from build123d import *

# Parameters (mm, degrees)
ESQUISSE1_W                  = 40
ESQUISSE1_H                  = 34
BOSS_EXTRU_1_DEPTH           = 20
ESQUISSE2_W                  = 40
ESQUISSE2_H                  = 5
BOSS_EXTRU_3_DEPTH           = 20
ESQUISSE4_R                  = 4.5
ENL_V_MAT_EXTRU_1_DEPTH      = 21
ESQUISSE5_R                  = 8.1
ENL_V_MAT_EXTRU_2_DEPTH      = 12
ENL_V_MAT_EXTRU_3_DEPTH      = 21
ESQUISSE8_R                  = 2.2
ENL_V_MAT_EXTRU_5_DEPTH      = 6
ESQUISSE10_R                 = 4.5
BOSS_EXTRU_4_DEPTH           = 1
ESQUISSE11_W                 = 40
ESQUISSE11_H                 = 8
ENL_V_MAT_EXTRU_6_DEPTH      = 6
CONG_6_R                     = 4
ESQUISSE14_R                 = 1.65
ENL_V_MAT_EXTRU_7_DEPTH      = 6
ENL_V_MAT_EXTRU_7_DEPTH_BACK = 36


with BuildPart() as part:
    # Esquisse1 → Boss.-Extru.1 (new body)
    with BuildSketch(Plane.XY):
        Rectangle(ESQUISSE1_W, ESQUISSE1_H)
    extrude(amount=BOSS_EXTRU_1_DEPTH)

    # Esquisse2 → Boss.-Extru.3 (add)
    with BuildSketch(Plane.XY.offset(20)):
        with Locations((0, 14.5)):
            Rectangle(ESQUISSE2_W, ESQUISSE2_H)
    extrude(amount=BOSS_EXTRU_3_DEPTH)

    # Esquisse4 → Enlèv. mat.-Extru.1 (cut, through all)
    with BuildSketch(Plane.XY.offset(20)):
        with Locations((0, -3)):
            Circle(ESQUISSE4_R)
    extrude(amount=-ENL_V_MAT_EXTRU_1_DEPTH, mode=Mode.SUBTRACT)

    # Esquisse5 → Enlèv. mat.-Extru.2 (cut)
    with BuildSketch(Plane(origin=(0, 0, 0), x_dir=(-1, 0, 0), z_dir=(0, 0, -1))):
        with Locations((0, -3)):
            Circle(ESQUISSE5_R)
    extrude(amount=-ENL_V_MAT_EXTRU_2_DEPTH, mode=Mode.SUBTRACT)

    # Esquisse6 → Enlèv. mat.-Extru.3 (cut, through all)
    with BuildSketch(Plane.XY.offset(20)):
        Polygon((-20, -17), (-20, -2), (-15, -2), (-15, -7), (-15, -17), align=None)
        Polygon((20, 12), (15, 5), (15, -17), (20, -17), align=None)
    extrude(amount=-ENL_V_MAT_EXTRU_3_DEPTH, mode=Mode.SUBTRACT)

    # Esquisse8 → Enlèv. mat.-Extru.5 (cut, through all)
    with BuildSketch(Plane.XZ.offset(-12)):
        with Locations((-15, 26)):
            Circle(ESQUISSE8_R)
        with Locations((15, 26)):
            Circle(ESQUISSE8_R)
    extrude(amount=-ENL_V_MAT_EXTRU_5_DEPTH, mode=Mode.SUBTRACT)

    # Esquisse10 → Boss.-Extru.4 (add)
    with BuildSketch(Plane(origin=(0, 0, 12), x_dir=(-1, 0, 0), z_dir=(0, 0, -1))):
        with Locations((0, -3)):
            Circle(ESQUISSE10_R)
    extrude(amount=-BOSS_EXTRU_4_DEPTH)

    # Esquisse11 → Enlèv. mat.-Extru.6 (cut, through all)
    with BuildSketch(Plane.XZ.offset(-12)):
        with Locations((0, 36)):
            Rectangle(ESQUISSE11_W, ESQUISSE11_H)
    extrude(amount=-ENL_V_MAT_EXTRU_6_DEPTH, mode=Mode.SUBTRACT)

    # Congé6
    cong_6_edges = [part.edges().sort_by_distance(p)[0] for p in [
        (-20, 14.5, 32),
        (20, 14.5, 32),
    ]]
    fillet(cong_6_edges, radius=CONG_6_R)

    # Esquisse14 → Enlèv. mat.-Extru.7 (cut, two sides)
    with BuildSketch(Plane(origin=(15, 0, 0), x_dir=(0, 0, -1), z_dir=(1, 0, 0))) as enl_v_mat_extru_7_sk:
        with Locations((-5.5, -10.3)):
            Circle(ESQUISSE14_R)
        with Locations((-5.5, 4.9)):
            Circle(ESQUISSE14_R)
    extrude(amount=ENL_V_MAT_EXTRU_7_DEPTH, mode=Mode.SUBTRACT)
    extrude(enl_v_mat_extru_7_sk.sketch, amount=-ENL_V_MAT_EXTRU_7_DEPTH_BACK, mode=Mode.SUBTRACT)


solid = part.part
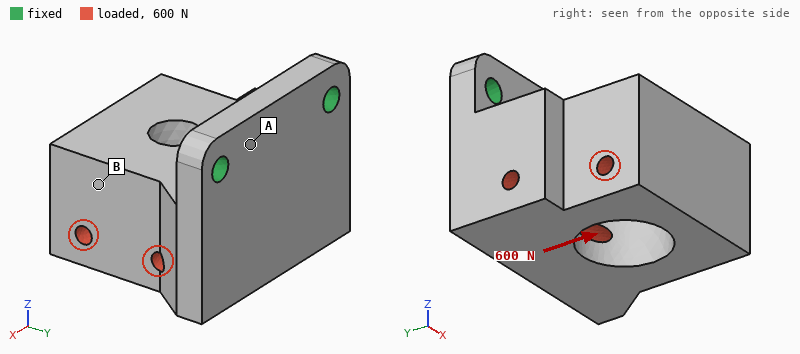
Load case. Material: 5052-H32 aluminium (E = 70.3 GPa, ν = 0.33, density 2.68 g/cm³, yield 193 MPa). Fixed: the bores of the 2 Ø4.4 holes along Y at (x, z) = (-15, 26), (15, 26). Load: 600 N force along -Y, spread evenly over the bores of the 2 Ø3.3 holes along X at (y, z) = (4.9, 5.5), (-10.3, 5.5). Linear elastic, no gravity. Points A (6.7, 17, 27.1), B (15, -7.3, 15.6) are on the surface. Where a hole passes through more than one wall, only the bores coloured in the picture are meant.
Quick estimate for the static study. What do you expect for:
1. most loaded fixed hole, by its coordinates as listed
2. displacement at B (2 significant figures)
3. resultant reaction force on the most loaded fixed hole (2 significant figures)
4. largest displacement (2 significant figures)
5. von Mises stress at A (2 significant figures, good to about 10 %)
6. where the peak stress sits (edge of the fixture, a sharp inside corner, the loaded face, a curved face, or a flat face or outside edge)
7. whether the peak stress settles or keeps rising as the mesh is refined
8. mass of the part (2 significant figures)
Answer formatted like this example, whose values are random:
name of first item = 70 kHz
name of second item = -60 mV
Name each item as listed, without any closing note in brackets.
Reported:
most loaded fixed hole, by its coordinates as listed = (-15, 26)
displacement at B = 0.070 mm
resultant reaction force on the most loaded fixed hole = 330 N
largest displacement = 0.12 mm
von Mises stress at A = 22 MPa
where the peak stress sits = edge of the fixture
whether the peak stress settles or keeps rising as the mesh is refined = keeps rising
mass of the part = 59 g
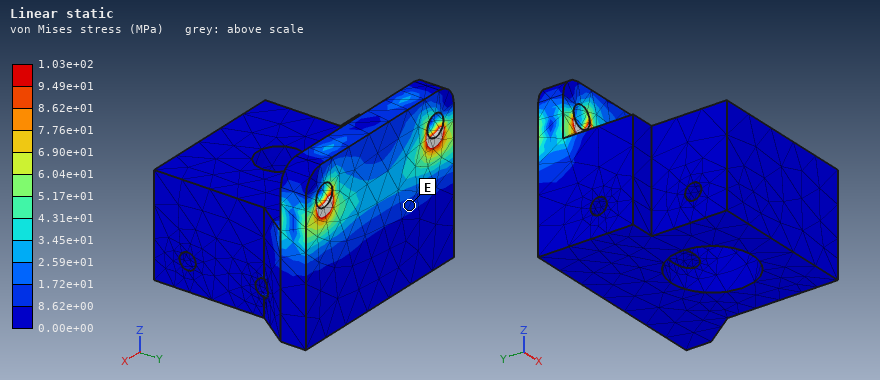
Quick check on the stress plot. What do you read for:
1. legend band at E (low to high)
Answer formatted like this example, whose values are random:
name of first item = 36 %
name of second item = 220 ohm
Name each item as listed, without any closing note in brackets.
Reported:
legend band at E = 8.62e+00 to 1.72e+01 MPa
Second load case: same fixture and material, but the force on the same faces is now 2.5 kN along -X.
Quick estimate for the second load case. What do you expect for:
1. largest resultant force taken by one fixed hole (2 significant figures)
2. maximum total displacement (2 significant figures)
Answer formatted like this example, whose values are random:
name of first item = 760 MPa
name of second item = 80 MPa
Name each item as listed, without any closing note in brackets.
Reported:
largest resultant force taken by one fixed hole = 2.4 kN
maximum total displacement = 45 µm
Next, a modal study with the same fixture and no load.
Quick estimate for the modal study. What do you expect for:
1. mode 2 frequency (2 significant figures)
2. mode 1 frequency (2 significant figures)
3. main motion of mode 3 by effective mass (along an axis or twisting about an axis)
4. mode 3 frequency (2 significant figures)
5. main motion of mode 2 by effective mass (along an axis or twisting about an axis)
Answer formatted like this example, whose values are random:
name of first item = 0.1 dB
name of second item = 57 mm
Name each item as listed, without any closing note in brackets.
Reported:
mode 2 frequency = 6600 Hz
mode 1 frequency = 1900 Hz
main motion of mode 3 by effective mass = along Y
mode 3 frequency = 11 kHz
main motion of mode 2 by effective mass = along X
